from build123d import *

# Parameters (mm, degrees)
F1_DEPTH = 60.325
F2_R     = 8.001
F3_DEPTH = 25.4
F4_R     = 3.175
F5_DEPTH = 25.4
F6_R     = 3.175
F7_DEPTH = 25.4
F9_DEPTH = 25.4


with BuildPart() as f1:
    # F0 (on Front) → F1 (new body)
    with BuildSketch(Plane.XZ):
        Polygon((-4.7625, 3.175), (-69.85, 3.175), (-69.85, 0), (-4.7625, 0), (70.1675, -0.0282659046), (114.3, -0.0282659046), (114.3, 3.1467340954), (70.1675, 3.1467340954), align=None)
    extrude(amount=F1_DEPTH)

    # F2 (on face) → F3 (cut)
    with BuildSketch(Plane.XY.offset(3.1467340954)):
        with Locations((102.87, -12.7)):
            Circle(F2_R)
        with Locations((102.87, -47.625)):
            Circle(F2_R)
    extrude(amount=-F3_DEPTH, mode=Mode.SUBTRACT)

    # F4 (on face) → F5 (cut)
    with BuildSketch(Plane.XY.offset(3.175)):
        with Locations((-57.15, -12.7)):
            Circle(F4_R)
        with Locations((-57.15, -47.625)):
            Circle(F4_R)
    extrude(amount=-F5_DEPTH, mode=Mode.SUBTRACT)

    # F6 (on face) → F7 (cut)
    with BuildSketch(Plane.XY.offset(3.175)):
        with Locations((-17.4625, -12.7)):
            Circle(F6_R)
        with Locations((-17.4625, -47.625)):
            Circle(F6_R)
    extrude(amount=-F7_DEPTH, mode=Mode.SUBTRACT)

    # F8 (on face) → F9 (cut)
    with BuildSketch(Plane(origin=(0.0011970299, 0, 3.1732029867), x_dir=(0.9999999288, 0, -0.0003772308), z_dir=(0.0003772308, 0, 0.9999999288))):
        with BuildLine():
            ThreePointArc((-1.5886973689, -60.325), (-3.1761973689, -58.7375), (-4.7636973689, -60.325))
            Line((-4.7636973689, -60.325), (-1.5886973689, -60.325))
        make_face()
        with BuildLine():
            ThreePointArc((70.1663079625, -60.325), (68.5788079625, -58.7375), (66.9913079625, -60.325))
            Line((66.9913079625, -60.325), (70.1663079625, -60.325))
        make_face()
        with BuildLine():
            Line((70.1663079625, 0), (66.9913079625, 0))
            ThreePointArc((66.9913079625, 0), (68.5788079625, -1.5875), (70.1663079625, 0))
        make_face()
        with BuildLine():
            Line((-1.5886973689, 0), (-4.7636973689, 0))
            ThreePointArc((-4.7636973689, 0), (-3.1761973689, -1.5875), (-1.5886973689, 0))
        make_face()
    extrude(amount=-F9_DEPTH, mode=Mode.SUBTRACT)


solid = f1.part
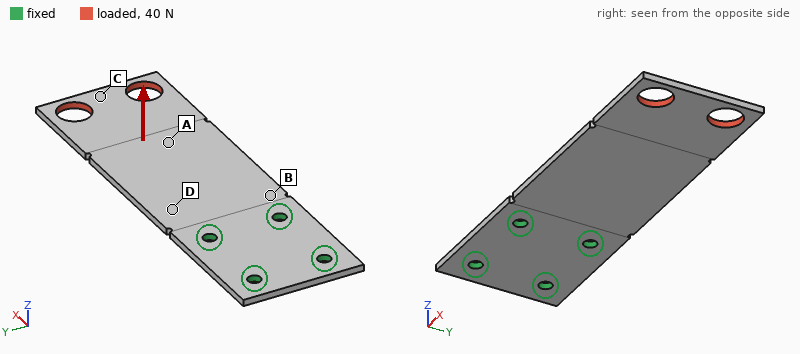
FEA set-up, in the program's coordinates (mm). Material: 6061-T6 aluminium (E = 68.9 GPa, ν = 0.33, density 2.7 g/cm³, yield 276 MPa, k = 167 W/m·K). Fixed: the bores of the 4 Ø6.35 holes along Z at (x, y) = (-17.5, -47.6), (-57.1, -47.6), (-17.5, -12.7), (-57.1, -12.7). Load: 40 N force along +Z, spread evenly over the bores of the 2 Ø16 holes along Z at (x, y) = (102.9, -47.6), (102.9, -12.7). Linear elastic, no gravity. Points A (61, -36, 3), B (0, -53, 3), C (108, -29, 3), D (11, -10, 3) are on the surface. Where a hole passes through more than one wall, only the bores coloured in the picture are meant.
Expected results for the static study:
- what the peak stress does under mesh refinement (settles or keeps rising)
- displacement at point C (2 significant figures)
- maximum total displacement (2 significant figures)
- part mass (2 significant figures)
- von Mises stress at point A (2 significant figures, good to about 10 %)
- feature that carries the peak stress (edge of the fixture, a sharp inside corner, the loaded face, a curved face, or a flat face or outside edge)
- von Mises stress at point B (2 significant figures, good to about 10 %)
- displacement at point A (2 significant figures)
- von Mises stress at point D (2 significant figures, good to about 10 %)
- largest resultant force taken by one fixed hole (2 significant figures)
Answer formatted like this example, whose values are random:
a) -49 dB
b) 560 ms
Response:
a) keeps rising
b) 2.1 mm
c) 2.3 mm
d) 91 g
e) 17 MPa
f) edge of the fixture
g) 41 MPa
h) 0.99 mm
i) 35 MPa
j) 27 N
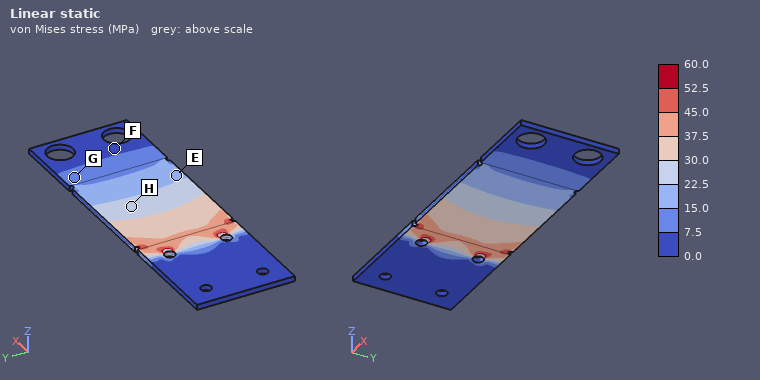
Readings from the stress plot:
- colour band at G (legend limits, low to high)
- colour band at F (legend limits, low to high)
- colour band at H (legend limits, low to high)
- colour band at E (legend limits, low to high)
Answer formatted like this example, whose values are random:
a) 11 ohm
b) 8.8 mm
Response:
a) 7.5 to 15.0 MPa
b) 0.0 to 7.5 MPa
c) 22.5 to 30.0 MPa
d) 15.0 to 22.5 MPa
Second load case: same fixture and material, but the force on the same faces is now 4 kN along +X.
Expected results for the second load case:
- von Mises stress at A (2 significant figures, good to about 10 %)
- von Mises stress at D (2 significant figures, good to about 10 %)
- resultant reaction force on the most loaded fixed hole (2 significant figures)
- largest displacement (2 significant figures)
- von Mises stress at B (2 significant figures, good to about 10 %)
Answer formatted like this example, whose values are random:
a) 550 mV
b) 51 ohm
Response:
a) 20 MPa
b) 21 MPa
c) 1.8 kN
d) 76 µm
e) 21 MPa
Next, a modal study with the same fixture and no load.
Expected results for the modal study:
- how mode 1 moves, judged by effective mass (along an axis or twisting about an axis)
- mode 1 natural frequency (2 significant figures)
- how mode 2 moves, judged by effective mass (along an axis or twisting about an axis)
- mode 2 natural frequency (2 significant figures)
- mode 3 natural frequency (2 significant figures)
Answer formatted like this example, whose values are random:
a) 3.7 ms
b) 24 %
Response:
a) along Z
b) 170 Hz
c) twisting about X
d) 730 Hz
e) 1000 Hz
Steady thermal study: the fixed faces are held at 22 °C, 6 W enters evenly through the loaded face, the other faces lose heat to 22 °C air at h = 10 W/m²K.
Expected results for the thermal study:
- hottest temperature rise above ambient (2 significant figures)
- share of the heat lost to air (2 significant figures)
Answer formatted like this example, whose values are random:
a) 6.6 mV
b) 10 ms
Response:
a) 21 K
b) 26 %
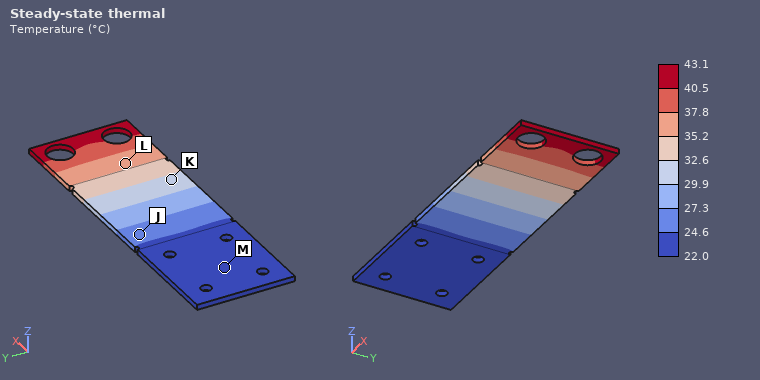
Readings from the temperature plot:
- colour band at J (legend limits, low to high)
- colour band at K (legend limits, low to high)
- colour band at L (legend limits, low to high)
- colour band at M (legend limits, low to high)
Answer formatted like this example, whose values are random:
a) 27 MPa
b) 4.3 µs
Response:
a) 24.6 to 27.3 °C
b) 29.9 to 32.6 °C
c) 35.2 to 37.8 °C
d) 22.0 to 24.6 °C
